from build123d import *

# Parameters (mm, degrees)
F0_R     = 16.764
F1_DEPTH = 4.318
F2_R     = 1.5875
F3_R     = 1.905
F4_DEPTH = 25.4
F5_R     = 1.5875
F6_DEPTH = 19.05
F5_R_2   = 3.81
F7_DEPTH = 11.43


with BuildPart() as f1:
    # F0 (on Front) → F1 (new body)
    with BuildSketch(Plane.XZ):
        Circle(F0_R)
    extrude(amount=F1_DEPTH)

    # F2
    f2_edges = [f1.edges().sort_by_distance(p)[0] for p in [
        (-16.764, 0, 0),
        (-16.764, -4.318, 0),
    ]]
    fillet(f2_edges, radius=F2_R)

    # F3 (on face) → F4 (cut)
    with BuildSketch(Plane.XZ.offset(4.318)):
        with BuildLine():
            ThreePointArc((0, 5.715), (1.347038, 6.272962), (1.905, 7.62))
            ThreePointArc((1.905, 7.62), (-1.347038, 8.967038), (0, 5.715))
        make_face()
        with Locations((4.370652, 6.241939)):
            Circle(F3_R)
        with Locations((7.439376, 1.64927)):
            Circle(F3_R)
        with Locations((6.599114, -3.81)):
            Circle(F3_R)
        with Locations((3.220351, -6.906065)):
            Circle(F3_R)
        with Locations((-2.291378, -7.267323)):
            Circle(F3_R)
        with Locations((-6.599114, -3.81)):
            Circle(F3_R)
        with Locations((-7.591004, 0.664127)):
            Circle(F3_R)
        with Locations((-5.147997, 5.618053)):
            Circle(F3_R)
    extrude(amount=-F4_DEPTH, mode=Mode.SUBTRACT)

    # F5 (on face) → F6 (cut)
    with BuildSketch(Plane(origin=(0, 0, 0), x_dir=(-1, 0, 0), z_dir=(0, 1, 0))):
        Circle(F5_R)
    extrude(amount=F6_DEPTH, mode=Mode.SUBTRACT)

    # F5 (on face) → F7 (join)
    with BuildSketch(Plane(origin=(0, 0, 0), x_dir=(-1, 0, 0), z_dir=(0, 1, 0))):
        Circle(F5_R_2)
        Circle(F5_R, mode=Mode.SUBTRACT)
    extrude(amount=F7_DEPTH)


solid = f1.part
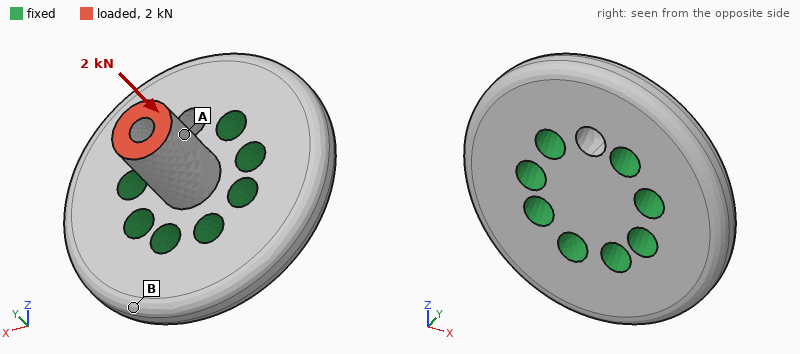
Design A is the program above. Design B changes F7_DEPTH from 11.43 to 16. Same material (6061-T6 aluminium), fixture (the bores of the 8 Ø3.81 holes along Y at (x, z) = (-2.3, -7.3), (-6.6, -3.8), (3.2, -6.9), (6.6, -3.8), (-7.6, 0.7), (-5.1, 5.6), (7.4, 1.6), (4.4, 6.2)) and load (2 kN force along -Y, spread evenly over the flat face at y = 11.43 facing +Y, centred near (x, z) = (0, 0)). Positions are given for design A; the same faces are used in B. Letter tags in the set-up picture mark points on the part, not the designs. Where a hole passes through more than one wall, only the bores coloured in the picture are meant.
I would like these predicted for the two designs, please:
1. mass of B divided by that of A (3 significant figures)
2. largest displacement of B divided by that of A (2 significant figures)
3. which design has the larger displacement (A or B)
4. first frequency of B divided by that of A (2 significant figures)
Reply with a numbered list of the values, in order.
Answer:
1. 1.05
2. 1.3
3. B
4. 0.59
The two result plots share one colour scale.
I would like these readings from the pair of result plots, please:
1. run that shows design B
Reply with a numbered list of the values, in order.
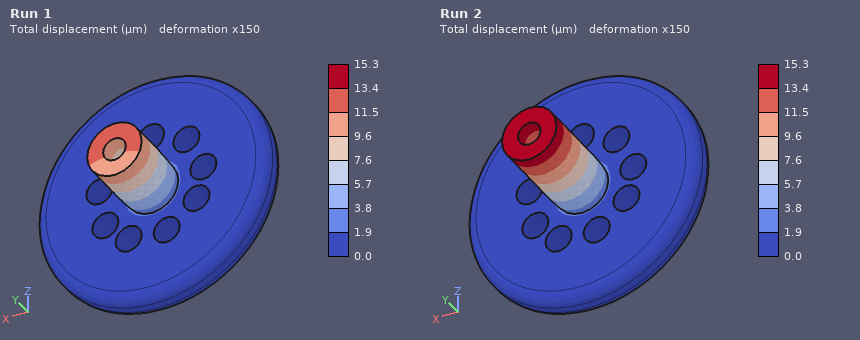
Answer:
1. Run 2
